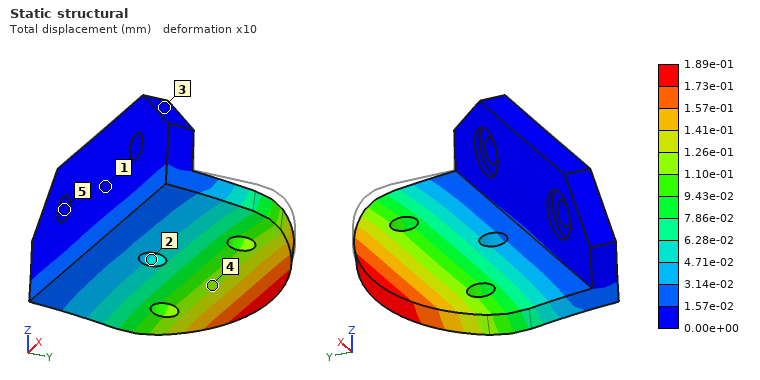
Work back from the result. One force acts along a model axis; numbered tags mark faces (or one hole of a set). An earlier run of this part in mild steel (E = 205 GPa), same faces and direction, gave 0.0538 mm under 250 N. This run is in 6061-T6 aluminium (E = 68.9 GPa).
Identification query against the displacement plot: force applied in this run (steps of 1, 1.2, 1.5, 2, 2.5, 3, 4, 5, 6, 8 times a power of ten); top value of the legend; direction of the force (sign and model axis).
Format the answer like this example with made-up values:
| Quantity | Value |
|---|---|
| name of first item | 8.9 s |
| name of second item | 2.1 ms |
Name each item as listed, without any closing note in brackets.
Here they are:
| Quantity | Value |
|---|---|
| force applied in this run | 300 N |
| top value of the legend | 1.89e-01 mm |
| direction of the force | -Z |
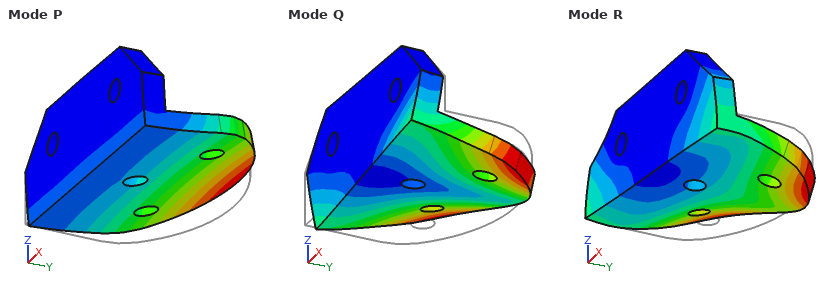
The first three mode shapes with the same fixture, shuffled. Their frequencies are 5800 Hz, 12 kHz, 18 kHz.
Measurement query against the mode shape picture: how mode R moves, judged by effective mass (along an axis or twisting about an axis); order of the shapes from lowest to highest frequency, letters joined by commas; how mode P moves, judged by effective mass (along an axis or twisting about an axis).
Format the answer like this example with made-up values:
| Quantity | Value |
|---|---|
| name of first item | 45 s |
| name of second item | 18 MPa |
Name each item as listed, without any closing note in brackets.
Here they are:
| Quantity | Value |
|---|---|
| how mode R moves, judged by effective mass | along X |
| order of the shapes from lowest to highest frequency, letters joined by commas | P, Q, R |
| how mode P moves, judged by effective mass | along Z |
